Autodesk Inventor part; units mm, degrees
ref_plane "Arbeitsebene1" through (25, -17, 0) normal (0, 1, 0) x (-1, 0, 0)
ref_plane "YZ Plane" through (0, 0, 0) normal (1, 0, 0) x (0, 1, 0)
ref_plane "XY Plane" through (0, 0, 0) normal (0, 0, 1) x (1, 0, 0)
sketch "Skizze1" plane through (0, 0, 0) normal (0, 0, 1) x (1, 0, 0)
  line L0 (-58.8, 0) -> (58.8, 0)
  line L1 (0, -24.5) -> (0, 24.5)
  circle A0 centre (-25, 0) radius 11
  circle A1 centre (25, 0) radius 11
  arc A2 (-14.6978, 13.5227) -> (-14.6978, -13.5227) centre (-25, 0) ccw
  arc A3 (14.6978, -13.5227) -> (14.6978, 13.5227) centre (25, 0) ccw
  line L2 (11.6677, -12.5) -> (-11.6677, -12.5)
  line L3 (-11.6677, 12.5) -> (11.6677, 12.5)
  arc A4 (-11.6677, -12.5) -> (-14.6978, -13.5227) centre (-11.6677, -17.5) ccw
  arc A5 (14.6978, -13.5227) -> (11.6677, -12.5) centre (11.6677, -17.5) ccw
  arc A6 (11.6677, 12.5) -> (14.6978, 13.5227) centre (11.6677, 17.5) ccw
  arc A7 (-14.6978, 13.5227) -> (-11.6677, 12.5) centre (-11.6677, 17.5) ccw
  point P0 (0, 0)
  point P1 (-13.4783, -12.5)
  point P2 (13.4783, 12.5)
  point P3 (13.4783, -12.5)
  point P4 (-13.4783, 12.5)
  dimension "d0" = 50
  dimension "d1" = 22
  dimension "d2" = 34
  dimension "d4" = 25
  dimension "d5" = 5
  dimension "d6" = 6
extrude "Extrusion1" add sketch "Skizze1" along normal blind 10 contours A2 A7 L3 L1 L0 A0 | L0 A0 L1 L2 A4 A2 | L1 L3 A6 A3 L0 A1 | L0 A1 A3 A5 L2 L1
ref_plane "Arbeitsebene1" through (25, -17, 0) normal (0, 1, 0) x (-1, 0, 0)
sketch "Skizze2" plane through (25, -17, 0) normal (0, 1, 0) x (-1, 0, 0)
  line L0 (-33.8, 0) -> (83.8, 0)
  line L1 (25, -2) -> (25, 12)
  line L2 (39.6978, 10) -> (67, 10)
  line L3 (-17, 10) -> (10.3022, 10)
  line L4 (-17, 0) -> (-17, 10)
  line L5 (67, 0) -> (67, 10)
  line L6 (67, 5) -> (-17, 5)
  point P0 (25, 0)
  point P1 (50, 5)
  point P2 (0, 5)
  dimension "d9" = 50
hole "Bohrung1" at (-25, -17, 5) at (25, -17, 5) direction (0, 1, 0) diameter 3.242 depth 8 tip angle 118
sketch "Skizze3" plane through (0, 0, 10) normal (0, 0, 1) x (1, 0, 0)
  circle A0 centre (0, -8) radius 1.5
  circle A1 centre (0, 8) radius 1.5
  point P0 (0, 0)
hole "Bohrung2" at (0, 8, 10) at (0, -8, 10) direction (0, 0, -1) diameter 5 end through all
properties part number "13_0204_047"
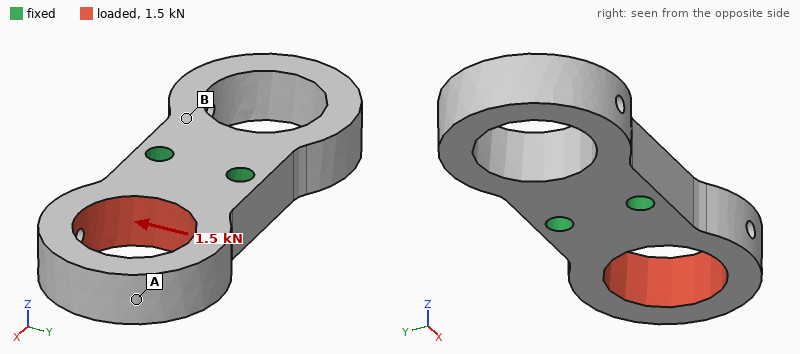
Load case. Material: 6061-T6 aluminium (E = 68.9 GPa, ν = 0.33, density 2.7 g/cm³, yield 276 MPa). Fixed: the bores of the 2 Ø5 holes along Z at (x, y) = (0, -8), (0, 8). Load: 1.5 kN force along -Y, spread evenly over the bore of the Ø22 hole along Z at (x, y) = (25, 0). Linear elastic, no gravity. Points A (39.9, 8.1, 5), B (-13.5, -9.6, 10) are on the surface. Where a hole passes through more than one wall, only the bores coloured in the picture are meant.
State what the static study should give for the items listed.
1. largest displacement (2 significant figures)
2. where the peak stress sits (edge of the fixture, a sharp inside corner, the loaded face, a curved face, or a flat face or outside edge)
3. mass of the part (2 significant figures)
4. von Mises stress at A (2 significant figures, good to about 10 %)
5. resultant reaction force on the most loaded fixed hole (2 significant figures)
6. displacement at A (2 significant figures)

76 µm
a curved face
40 g
23 MPa
2.1 kN
75 µm
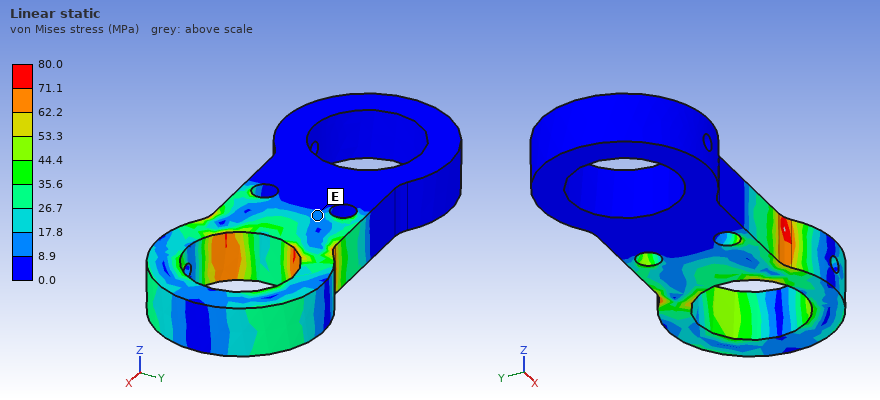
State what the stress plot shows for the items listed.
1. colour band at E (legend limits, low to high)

8.9 to 17.8 MPa
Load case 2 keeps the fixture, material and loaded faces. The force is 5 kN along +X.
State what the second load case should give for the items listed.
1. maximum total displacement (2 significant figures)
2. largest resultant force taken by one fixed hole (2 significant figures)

39 µm
2.5 kN
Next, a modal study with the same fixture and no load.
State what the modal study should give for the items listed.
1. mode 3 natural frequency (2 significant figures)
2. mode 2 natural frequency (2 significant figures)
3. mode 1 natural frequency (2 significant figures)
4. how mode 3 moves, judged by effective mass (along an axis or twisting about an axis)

6500 Hz
4800 Hz
4600 Hz
twisting about Z
